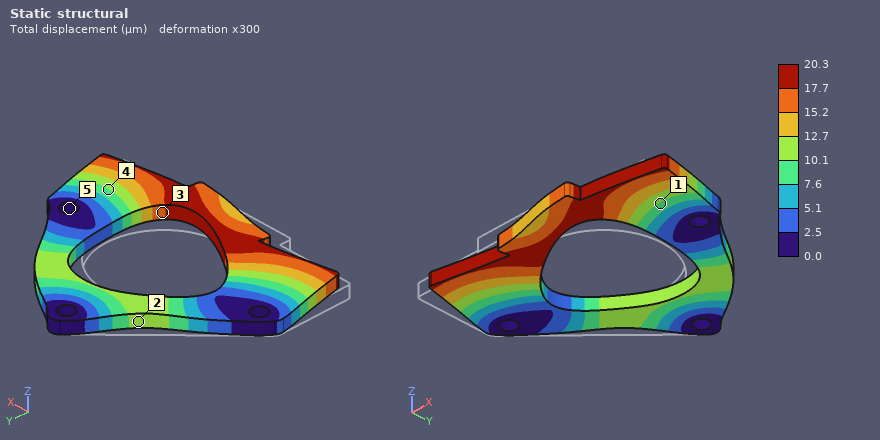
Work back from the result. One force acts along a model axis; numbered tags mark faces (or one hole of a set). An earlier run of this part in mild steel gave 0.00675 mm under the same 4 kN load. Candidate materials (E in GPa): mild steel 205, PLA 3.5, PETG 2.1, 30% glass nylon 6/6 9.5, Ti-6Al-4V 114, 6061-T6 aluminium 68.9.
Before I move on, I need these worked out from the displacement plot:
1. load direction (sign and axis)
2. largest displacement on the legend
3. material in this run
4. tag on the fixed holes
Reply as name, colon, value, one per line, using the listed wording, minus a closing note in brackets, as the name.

load direction: +X
largest displacement on the legend: 20.3 µm
material in this run: 6061-T6 aluminium
tag on the fixed holes: 5
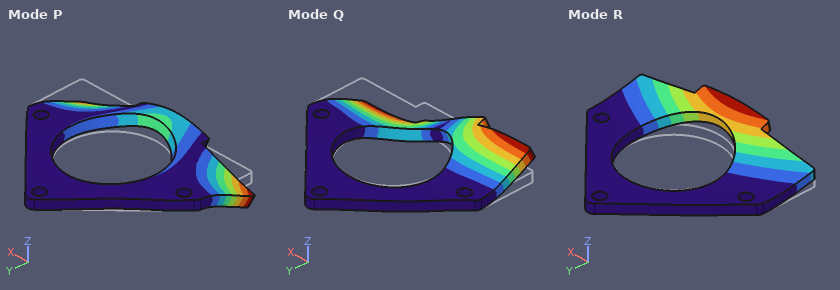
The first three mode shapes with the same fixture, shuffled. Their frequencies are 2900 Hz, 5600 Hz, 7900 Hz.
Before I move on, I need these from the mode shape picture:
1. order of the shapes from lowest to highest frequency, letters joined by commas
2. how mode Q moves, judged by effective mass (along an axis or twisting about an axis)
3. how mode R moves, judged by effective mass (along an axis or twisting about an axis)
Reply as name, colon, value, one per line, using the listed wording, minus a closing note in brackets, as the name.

order of the shapes from lowest to highest frequency, letters joined by commas: R, Q, P
how mode Q moves, judged by effective mass: twisting about Y
how mode R moves, judged by effective mass: along Z
